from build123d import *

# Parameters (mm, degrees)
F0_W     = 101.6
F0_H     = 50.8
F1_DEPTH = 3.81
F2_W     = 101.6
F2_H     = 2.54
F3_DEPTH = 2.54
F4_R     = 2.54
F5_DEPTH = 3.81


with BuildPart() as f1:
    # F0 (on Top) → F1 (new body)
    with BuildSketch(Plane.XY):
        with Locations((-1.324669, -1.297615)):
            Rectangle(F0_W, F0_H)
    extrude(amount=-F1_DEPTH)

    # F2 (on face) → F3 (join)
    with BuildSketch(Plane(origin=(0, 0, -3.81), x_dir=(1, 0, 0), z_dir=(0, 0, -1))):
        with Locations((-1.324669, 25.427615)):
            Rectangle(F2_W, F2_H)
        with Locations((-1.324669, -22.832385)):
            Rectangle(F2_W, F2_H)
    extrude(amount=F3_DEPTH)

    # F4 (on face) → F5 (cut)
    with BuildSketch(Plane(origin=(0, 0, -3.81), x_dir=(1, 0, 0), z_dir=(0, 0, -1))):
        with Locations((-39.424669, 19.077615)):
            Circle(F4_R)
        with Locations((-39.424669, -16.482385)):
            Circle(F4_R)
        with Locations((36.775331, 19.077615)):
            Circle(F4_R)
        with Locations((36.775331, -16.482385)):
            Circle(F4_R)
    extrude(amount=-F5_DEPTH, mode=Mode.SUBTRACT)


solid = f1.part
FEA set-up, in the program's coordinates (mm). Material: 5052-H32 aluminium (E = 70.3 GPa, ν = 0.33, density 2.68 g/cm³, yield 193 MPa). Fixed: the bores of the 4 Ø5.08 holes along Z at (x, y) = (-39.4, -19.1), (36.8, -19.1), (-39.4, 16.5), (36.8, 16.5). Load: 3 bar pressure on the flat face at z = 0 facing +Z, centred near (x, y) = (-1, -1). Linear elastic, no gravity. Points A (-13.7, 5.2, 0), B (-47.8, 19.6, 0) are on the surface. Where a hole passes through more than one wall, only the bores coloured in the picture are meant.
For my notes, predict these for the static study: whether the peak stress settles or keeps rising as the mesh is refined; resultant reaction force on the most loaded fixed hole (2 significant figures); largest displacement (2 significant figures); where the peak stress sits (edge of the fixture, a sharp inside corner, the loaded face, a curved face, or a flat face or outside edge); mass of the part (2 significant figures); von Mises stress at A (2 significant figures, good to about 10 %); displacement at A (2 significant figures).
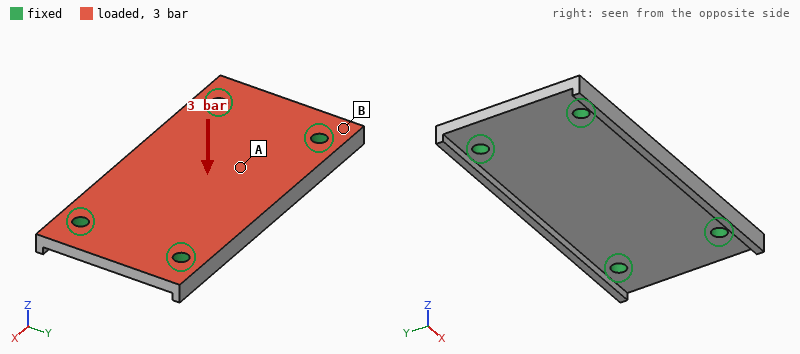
keeps rising
390 N
64 µm
edge of the fixture
55 g
15 MPa
52 µm
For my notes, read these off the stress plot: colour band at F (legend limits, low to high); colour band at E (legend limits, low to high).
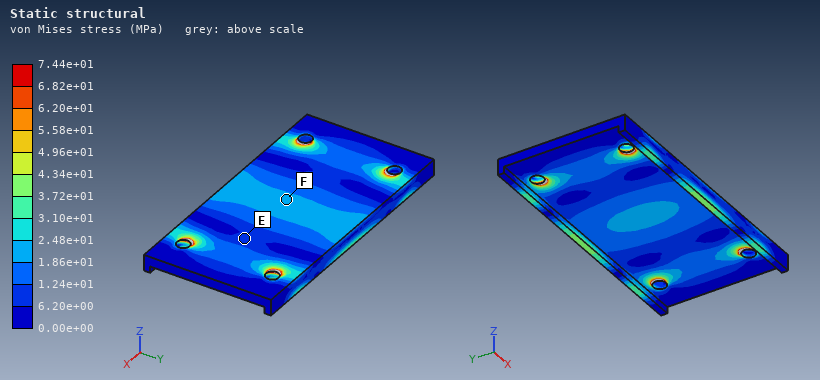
1.86e+01 to 2.48e+01 MPa
6.20e+00 to 1.24e+01 MPa
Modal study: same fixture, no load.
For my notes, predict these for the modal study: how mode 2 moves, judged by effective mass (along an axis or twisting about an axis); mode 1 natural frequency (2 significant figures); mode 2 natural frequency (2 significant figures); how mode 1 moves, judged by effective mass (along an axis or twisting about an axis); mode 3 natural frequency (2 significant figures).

twisting about X
3800 Hz
5300 Hz
along Z
9800 Hz
